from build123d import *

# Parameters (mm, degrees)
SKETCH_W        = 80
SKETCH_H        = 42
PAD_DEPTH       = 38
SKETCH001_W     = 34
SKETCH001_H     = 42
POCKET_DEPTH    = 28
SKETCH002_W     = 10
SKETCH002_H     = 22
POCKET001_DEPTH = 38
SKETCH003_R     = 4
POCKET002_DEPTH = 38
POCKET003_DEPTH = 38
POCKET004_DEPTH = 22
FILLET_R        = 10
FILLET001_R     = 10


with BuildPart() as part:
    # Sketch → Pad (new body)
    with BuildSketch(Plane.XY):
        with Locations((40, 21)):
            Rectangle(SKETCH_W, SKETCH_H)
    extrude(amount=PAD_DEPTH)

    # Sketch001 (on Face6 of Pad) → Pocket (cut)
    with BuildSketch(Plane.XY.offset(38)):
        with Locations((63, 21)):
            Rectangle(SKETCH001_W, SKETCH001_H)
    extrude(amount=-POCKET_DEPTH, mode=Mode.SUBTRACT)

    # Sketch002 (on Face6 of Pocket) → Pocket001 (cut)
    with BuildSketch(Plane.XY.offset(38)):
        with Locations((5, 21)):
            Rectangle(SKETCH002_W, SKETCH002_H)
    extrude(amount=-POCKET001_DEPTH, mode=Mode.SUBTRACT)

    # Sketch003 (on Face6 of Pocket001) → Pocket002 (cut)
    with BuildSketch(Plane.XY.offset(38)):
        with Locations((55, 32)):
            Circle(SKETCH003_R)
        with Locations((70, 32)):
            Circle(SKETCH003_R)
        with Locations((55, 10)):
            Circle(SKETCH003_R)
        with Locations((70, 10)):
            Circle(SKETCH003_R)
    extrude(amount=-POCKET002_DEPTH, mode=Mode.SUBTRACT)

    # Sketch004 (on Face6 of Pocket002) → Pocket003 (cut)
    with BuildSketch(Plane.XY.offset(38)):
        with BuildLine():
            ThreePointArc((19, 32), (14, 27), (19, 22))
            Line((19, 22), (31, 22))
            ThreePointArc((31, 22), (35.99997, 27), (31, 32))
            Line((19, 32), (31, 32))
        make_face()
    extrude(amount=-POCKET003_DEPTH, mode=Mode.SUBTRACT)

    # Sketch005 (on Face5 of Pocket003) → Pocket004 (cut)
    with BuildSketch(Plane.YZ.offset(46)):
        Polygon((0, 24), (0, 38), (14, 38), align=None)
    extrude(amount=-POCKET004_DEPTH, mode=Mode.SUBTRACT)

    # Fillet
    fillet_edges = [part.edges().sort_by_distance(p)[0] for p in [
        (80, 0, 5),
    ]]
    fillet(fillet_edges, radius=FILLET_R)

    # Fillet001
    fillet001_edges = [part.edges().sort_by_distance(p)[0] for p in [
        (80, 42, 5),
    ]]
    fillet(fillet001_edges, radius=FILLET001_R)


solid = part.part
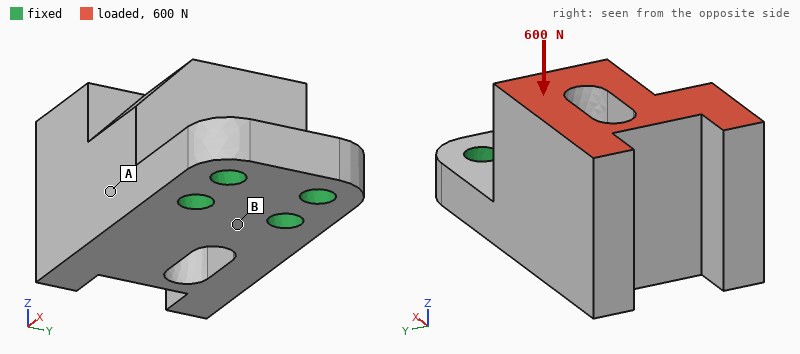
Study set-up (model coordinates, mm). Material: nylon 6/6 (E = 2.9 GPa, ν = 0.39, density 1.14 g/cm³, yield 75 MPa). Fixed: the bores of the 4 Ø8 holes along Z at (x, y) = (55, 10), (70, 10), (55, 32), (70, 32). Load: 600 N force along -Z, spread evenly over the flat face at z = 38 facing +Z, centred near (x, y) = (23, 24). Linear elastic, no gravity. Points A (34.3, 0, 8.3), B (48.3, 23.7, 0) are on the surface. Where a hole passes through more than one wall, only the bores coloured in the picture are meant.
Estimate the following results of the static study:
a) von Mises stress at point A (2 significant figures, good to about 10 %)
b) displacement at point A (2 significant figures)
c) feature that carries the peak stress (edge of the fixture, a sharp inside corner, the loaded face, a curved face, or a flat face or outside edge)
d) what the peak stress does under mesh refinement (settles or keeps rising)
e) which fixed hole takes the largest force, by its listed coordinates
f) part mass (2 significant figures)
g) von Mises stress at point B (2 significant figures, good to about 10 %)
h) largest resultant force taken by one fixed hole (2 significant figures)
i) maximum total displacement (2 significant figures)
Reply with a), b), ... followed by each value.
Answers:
a) 3.3 MPa
b) 0.24 mm
c) edge of the fixture
d) keeps rising
e) (55, 32)
f) 77 g
g) 14 MPa
h) 430 N
i) 1.0 mm
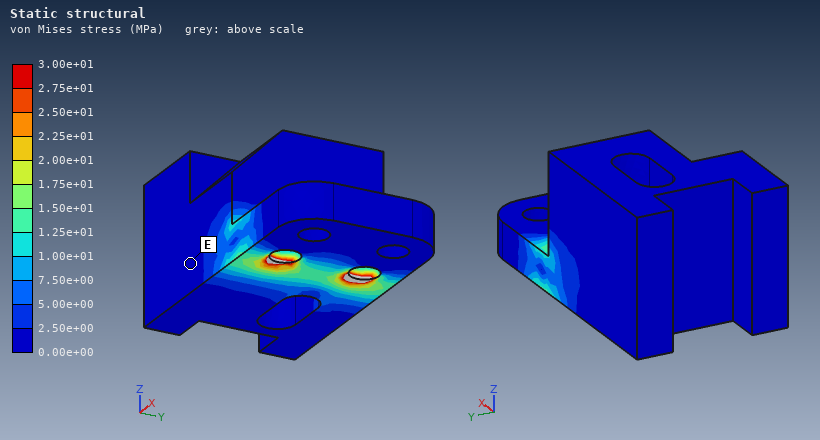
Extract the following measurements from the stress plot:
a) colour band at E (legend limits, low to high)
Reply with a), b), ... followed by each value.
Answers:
a) 0.00e+00 to 2.50e+00 MPa
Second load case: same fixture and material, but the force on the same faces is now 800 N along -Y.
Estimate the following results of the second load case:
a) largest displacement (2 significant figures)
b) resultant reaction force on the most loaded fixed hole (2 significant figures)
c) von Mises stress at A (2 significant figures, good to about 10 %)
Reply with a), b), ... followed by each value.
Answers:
a) 0.45 mm
b) 1.3 kN
c) 2.8 MPa
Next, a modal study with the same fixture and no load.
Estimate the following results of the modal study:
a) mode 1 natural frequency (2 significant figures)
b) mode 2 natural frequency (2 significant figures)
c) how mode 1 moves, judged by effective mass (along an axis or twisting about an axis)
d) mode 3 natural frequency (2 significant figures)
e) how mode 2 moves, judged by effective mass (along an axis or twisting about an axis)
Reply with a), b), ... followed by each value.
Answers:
a) 590 Hz
b) 1500 Hz
c) along Z
d) 1900 Hz
e) along Y
